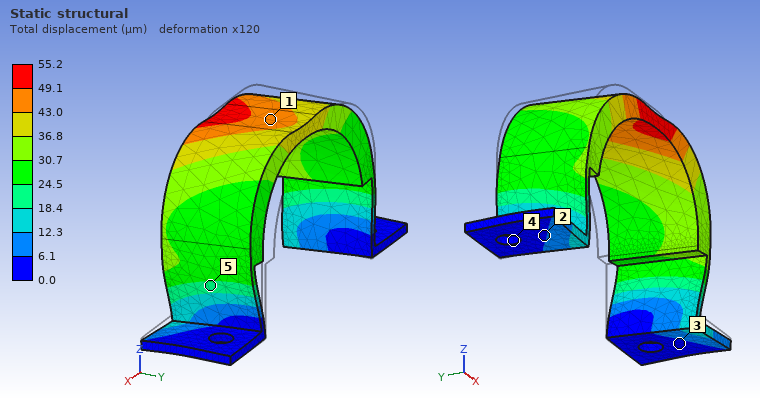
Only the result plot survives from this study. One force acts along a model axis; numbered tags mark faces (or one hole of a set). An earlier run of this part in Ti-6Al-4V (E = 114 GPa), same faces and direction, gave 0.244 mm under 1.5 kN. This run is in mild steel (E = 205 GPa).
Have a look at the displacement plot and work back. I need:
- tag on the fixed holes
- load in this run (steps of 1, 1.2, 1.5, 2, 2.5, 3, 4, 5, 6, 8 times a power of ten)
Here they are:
4
600 N
